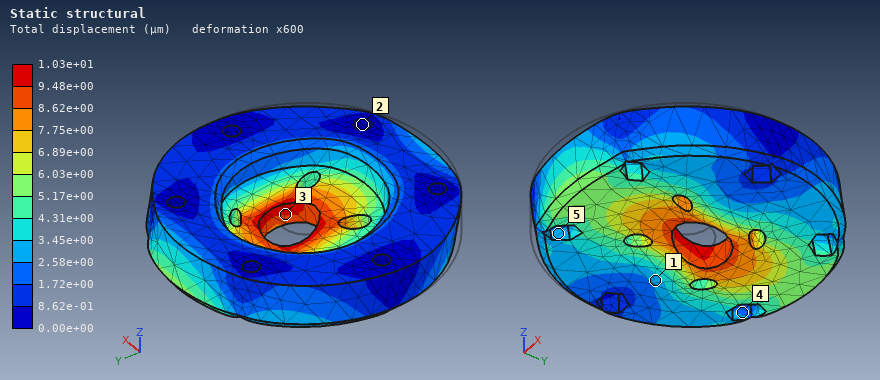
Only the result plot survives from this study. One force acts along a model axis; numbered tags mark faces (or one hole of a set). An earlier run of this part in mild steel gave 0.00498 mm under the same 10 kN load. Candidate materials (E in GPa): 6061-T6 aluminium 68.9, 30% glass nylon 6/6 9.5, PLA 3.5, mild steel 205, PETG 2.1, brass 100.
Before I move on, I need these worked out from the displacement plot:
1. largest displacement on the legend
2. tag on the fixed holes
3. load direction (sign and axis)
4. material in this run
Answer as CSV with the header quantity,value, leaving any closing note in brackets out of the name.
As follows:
quantity,value
largest displacement on the legend,1.03e+01 µm
tag on the fixed holes,2
load direction,+Y
material in this run,brass
